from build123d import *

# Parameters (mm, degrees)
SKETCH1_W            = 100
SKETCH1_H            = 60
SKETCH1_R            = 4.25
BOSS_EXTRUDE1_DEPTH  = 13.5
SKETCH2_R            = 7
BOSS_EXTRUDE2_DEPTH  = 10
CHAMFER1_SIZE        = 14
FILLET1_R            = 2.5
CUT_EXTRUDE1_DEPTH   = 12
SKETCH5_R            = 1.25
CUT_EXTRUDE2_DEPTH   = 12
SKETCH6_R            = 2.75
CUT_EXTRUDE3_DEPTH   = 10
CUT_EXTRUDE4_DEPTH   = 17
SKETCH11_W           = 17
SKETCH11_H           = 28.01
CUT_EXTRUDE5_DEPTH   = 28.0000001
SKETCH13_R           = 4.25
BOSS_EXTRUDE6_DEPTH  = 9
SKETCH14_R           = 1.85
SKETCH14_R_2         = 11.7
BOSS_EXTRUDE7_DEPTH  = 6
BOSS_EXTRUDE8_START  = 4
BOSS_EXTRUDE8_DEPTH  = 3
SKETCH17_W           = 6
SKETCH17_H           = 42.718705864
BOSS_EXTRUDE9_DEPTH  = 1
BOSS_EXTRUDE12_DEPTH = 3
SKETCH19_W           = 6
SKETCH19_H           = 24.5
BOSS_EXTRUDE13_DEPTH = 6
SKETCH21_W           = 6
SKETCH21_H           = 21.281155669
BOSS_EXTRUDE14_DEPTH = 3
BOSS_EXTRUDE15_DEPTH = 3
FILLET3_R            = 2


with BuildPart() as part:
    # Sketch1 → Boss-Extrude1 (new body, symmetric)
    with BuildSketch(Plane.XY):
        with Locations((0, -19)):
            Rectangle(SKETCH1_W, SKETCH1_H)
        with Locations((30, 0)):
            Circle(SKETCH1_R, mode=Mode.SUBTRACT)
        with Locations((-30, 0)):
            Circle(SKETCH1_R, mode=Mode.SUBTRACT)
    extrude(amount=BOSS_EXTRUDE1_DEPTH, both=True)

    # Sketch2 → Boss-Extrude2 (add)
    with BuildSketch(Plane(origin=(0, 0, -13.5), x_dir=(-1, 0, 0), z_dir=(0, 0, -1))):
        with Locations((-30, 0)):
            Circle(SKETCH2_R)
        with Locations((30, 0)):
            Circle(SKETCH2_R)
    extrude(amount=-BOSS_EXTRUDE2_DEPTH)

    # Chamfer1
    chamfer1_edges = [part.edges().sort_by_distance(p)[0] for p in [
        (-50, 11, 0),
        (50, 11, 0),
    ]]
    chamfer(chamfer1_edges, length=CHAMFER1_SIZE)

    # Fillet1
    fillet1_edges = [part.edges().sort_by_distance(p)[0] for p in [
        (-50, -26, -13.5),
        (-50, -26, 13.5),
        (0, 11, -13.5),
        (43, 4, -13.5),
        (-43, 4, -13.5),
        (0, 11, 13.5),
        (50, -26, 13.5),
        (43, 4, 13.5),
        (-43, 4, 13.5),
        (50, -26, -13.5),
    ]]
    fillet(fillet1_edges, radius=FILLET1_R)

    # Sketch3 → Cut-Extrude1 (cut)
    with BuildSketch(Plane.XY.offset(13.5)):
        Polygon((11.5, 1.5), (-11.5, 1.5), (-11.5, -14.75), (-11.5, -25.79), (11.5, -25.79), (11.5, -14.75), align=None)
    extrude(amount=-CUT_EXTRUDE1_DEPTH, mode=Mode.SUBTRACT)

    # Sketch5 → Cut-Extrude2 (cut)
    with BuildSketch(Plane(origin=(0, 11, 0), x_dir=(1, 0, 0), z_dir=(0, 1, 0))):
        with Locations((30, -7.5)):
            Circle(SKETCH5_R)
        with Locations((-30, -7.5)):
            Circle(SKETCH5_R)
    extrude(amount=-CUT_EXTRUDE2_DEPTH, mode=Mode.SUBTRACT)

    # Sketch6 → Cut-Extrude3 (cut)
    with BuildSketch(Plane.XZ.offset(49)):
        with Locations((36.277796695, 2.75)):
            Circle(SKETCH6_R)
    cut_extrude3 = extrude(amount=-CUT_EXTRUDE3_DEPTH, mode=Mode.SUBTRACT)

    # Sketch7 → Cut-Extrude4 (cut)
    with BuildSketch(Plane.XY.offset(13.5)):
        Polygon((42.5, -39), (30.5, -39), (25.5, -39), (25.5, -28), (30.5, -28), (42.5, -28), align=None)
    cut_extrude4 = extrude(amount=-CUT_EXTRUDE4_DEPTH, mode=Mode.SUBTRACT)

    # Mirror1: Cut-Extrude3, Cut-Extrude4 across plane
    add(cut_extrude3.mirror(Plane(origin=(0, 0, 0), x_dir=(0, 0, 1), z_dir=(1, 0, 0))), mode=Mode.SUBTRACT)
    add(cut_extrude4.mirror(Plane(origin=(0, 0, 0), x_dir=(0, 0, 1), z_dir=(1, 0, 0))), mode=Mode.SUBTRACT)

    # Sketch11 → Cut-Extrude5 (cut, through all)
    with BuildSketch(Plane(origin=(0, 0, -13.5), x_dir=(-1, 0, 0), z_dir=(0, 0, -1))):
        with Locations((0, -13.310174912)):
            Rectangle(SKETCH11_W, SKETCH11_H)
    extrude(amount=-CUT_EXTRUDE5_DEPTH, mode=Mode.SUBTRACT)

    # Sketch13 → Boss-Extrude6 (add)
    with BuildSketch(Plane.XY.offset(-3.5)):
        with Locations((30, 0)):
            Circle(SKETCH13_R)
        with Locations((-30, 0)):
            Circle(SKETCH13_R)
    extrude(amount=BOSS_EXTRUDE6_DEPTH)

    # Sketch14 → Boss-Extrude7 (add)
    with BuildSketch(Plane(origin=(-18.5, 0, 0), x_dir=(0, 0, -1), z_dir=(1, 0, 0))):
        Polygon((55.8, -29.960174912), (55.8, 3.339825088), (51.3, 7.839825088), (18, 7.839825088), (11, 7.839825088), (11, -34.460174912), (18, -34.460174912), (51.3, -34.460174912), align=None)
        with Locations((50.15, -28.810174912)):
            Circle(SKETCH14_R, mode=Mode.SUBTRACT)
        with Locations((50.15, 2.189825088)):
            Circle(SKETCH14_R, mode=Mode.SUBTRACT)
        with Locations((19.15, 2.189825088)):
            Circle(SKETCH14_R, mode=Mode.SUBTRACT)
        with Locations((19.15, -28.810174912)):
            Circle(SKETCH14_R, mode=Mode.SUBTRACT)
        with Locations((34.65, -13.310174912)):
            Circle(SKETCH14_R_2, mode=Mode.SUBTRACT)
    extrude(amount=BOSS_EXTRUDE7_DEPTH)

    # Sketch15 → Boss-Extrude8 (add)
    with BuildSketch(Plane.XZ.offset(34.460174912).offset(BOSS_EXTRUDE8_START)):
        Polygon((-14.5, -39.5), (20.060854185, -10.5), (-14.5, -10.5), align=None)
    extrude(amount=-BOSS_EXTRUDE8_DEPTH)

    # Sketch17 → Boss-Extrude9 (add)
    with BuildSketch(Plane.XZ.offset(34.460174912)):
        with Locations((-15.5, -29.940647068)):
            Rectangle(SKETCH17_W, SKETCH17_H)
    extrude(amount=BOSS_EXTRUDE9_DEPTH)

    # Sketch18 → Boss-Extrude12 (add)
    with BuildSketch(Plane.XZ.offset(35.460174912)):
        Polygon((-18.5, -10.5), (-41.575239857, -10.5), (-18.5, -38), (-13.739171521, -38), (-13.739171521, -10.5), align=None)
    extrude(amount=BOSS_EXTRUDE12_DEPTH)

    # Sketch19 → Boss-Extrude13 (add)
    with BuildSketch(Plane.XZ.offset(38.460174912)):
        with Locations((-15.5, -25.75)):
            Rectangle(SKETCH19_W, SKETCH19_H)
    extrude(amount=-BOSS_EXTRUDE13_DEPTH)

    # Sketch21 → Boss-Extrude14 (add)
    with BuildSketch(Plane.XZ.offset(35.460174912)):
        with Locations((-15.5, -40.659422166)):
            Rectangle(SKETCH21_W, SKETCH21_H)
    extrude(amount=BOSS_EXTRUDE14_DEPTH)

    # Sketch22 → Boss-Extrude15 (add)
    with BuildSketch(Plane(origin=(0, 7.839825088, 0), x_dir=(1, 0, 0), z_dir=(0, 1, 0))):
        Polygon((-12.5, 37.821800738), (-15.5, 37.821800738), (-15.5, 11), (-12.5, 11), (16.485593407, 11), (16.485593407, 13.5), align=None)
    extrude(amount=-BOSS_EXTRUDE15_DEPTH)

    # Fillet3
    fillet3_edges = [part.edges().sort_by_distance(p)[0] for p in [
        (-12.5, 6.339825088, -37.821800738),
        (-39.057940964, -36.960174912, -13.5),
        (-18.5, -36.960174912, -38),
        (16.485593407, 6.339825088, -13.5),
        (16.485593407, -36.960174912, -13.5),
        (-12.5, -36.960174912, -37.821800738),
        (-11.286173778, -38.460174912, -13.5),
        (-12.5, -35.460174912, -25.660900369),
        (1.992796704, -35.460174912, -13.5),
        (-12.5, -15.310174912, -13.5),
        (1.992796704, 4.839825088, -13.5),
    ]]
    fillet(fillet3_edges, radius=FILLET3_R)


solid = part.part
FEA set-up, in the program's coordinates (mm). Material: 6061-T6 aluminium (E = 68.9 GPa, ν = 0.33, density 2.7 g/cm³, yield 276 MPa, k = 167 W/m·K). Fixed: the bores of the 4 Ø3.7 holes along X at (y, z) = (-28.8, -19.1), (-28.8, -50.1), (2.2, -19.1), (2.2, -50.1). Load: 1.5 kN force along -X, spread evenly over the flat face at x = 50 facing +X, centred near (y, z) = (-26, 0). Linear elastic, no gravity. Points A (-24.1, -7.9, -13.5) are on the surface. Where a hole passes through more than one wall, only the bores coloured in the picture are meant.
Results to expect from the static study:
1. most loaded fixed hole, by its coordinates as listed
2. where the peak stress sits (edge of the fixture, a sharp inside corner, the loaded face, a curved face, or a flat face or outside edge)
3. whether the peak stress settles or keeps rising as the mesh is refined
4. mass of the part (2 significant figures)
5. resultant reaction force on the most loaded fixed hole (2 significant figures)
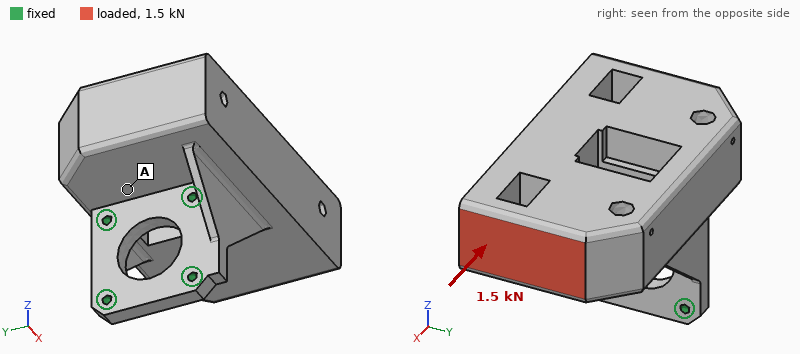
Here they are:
(-28.8, -19.1)
edge of the fixture
keeps rising
390 g
1.6 kN
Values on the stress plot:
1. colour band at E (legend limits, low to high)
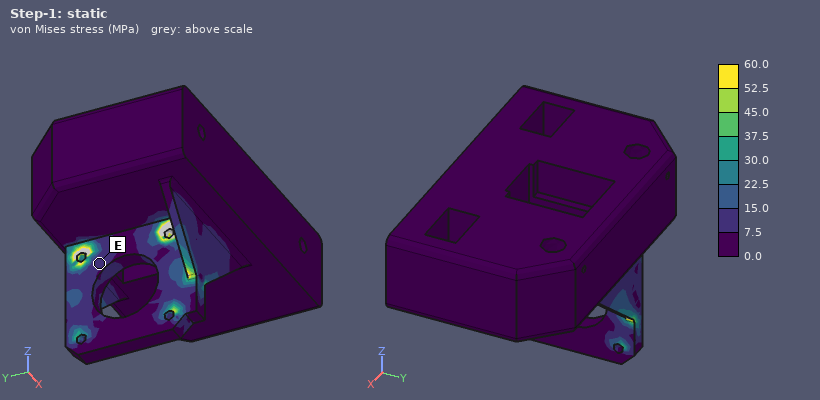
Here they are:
7.5 to 15.0 MPa
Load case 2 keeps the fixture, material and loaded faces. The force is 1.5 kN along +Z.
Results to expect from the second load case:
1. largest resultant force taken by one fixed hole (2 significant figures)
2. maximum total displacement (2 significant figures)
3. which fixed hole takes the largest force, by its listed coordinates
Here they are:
1.8 kN
0.33 mm
(-28.8, -19.1)
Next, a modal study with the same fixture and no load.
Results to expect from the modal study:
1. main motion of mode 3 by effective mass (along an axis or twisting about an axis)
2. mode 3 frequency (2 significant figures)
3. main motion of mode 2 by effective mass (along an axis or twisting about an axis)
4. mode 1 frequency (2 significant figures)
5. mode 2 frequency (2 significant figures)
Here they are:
along Y
4800 Hz
along Y
1000 Hz
2200 Hz
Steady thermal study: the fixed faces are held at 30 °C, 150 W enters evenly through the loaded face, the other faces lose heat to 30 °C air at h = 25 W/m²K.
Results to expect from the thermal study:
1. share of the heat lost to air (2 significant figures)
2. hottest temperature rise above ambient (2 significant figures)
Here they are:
17 %
81 K
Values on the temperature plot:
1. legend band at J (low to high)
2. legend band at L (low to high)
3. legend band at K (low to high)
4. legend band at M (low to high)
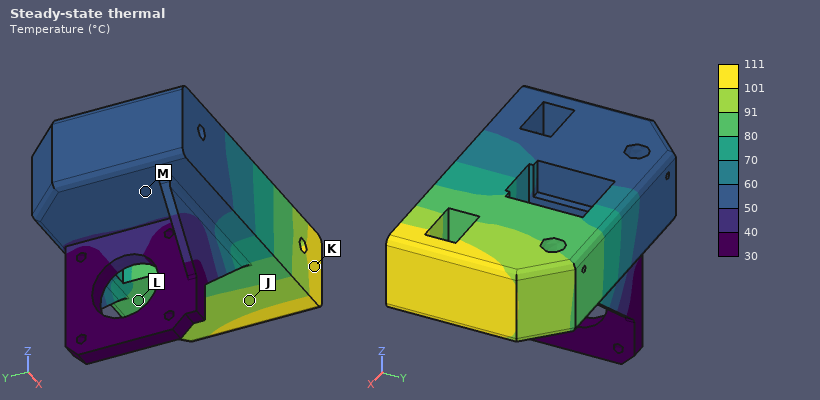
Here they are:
91 to 101 °C
80 to 91 °C
101 to 111 °C
50 to 60 °C
